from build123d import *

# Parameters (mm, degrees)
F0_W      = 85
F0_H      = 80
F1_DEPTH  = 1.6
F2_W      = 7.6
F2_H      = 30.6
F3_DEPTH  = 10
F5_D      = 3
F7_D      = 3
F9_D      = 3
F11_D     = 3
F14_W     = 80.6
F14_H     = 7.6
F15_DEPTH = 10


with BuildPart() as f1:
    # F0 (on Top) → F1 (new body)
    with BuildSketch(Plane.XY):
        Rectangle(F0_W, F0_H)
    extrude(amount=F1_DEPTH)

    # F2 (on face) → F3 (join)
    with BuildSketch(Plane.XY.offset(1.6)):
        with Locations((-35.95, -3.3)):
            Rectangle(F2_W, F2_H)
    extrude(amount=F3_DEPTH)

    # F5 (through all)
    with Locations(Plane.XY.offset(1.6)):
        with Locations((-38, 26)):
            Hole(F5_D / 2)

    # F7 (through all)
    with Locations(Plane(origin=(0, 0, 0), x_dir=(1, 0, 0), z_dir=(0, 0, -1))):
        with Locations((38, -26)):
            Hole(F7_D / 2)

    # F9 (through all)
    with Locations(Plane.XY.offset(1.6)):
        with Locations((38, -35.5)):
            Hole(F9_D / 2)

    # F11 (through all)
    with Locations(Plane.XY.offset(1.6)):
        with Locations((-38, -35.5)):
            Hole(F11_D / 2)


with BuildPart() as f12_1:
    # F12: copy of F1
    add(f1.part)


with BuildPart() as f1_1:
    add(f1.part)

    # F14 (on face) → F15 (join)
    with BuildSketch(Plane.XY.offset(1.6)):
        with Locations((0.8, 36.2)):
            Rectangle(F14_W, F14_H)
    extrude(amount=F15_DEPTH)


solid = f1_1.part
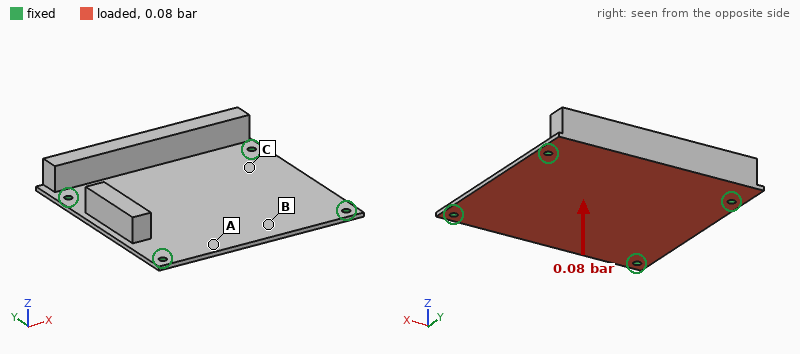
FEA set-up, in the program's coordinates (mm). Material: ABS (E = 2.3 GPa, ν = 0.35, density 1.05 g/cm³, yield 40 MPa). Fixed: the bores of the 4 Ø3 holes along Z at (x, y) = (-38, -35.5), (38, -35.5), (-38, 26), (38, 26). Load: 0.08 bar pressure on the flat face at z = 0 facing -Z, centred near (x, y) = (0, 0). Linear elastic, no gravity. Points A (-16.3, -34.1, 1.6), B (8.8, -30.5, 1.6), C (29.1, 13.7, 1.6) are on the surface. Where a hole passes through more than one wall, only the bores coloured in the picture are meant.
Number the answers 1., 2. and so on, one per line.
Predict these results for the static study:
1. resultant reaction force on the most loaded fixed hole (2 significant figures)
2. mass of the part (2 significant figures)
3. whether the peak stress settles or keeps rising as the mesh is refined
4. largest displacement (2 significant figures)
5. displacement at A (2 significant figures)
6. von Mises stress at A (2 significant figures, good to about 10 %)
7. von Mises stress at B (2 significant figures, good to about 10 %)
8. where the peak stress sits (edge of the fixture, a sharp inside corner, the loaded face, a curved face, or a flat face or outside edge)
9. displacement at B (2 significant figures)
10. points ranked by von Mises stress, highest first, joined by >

1. 18 N
2. 20 g
3. keeps rising
4. 1.2 mm
5. 0.79 mm
6. 3.1 MPa
7. 4.6 MPa
8. edge of the fixture
9. 1.1 mm
10. B > A > C
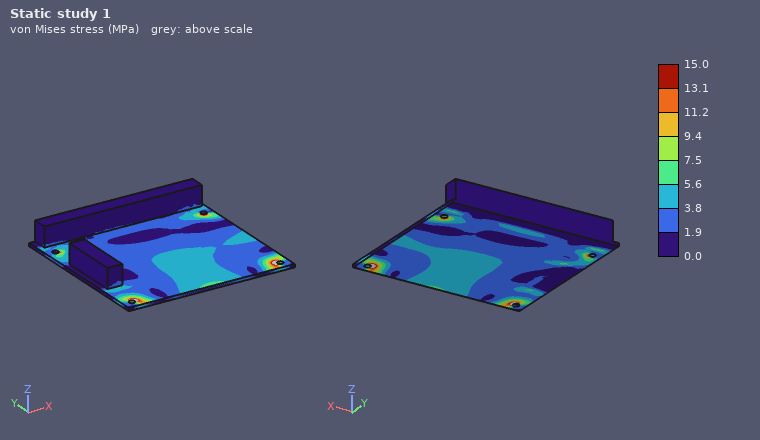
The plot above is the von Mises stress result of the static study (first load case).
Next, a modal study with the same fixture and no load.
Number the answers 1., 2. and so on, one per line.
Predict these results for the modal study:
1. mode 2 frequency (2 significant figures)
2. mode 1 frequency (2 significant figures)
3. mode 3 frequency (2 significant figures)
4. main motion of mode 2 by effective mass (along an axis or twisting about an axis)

1. 500 Hz
2. 350 Hz
3. 660 Hz
4. along Z
